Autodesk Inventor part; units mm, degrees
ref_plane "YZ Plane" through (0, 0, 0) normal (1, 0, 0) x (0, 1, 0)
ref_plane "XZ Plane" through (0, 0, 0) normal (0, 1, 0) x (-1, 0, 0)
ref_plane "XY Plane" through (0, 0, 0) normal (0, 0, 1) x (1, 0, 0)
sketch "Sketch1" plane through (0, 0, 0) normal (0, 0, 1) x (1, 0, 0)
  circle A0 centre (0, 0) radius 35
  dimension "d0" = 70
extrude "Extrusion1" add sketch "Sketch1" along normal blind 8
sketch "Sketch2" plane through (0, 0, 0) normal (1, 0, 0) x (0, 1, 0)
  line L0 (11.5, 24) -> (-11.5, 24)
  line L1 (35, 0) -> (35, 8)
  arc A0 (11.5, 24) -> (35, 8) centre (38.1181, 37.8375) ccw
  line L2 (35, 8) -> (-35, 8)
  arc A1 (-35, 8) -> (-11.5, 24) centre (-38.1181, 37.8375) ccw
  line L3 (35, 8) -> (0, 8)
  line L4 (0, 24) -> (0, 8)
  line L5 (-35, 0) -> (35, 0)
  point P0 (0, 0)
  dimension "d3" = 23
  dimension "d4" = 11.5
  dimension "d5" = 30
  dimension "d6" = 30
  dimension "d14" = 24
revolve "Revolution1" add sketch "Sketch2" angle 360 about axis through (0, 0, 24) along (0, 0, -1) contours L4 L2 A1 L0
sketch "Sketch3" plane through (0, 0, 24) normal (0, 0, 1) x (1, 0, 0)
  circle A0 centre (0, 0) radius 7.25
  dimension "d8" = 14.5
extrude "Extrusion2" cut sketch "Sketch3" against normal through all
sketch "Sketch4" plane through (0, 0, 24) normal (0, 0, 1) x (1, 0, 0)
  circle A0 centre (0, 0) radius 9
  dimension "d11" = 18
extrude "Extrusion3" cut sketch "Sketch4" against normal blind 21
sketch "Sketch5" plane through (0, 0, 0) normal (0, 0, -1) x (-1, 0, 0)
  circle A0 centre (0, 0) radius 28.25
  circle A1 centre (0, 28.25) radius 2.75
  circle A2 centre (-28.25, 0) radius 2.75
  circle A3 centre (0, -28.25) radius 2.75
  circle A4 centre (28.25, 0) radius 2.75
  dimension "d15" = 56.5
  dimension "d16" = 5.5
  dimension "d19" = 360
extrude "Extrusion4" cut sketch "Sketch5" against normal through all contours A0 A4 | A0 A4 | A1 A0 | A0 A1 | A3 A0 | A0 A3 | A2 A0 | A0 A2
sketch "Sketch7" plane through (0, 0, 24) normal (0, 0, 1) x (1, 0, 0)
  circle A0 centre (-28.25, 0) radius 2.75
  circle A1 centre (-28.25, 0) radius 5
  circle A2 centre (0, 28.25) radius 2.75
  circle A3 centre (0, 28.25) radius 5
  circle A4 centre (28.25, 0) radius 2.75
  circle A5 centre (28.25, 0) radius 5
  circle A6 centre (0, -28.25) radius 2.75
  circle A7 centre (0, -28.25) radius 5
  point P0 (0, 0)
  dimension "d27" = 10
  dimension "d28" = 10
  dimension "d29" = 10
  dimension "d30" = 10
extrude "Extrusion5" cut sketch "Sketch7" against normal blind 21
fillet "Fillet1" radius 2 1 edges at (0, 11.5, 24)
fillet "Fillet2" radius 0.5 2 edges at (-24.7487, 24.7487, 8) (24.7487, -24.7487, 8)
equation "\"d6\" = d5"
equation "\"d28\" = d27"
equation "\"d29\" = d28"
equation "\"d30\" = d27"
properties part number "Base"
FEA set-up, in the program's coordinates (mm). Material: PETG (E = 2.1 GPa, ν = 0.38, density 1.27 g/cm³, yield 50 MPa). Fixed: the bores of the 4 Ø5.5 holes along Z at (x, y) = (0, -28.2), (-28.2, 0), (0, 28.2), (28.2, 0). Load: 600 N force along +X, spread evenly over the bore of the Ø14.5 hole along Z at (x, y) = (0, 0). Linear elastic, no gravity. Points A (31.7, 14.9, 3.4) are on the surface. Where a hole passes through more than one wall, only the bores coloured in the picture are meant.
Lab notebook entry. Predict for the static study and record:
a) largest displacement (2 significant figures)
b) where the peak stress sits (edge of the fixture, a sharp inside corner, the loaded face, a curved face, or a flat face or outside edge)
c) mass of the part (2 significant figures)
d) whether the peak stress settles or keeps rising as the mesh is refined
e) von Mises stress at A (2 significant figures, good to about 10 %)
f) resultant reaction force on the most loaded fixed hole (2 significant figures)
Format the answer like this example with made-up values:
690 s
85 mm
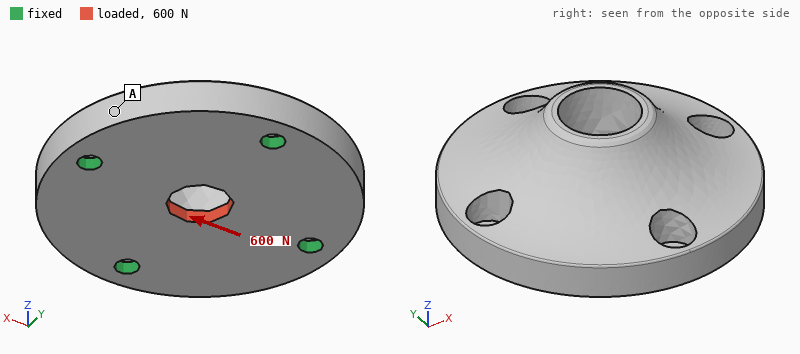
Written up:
33 µm
a sharp inside corner
54 g
keeps rising
0.68 MPa
170 N
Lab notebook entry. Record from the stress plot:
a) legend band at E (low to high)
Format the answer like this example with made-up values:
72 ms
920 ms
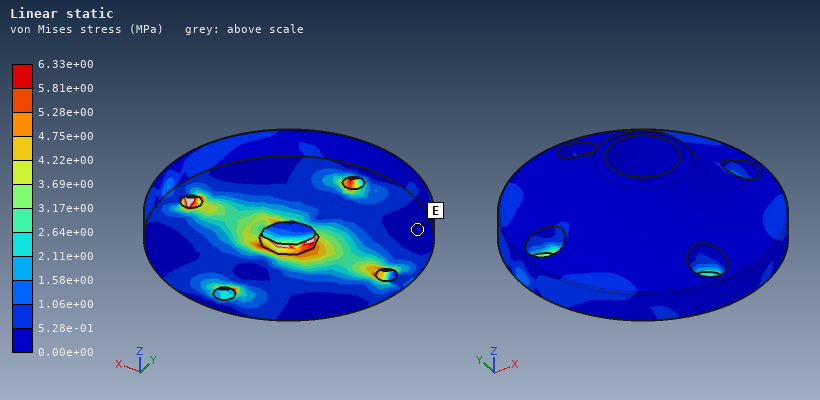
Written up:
0.00e+00 to 5.28e-01 MPa
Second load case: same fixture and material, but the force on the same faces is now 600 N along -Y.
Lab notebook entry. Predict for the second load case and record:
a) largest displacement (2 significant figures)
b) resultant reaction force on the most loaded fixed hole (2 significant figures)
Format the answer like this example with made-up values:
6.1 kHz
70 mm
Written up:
33 µm
170 N
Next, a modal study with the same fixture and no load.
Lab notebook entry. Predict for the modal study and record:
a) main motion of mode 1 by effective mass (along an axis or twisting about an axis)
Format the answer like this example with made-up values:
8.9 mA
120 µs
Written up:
along Z
